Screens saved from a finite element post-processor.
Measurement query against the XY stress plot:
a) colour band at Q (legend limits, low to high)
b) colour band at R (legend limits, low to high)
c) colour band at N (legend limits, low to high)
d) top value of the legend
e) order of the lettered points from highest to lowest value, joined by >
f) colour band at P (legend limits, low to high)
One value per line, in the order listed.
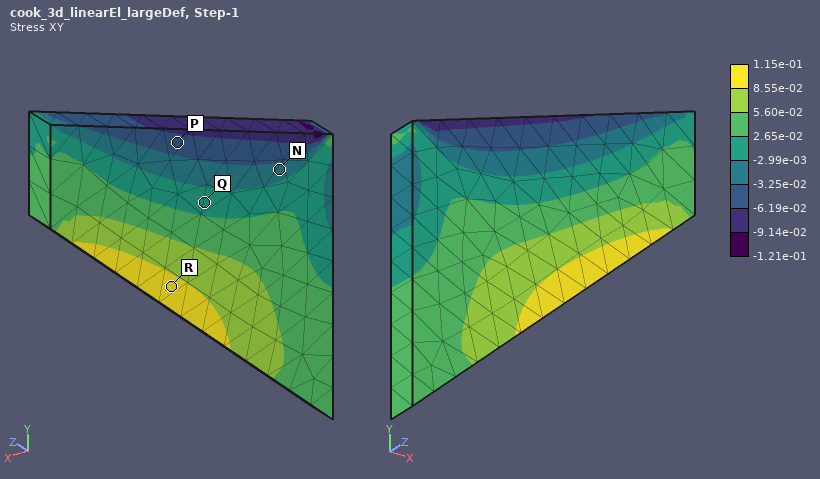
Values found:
-2.99e-03 to 2.65e-02
8.55e-02 to 1.15e-01
-3.25e-02 to -2.99e-03
1.15e-01
R > Q > N > P
-6.19e-02 to -3.25e-02
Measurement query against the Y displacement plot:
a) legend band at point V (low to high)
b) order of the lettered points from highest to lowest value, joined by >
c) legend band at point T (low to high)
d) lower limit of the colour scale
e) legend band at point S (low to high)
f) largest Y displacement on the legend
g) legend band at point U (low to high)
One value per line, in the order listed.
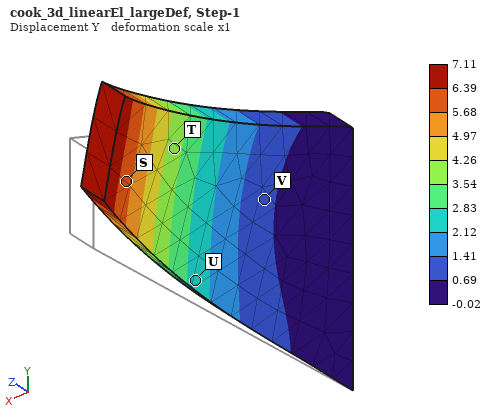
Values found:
0.69 to 1.41
S > T > U > V
3.54 to 4.26
-0.02
5.68 to 6.39
7.11
2.12 to 2.83
